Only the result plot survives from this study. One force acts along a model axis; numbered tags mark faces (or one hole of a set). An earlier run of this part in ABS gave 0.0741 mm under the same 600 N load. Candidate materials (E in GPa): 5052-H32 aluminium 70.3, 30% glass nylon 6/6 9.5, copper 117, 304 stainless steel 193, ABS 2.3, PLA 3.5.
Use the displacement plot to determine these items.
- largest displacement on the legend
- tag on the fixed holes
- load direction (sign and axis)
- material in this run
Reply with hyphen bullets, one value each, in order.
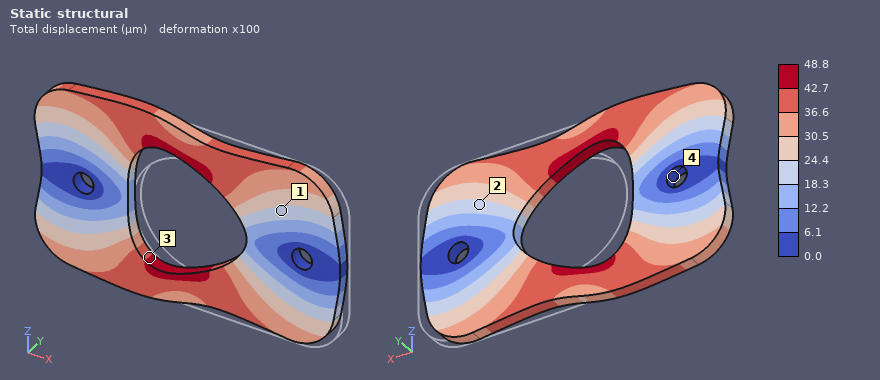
- 48.8 µm
- 4
- -X
- PLA
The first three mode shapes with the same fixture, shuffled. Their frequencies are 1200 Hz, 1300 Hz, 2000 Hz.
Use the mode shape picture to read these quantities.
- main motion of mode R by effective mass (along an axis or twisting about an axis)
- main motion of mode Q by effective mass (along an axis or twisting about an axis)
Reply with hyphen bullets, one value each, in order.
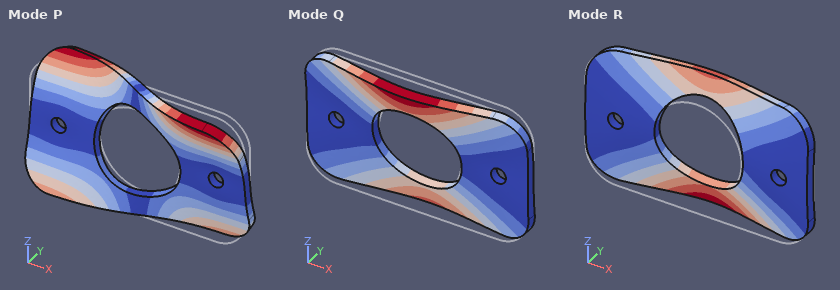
- along Y
- twisting about X
